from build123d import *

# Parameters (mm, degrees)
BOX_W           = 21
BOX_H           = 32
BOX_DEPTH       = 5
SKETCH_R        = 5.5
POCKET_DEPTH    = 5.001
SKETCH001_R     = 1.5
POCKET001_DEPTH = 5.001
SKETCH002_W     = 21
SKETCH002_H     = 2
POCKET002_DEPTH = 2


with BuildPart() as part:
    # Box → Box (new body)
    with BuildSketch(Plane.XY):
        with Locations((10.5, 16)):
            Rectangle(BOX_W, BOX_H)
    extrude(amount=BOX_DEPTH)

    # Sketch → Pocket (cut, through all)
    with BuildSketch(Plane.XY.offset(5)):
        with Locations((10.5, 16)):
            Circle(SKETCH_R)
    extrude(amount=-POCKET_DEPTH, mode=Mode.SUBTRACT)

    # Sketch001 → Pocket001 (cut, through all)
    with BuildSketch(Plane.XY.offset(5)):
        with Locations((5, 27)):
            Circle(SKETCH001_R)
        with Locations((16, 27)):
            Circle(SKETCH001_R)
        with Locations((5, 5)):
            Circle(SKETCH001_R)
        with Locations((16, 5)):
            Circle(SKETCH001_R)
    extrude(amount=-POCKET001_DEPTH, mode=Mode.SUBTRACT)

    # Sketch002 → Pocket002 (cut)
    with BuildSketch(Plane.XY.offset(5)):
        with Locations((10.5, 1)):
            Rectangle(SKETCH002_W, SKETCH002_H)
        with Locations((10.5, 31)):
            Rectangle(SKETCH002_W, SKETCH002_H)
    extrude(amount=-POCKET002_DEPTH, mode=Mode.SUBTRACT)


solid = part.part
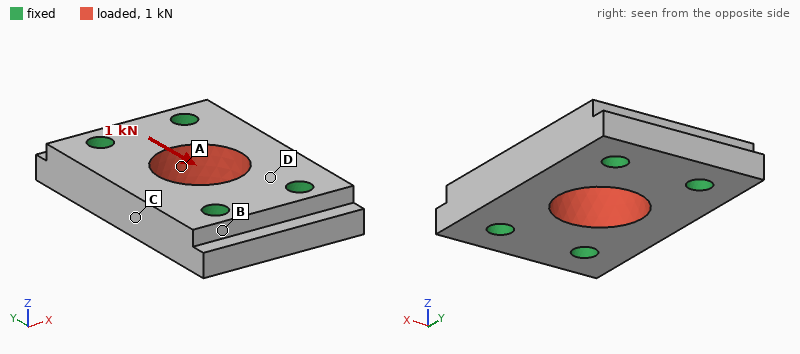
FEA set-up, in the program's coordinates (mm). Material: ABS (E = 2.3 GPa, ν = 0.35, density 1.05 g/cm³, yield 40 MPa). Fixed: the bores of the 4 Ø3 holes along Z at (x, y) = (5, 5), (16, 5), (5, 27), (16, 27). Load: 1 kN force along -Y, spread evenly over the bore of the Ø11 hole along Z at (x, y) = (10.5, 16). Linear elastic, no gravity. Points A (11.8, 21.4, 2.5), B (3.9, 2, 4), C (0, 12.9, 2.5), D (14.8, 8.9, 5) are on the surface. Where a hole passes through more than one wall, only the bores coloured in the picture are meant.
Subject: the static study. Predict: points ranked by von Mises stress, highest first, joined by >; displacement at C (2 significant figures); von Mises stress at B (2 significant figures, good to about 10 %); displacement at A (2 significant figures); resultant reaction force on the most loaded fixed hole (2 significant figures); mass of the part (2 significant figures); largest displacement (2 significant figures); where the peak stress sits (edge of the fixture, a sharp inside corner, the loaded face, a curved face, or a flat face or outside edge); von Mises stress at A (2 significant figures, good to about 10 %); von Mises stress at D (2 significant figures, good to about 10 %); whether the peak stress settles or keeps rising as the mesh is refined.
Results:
D > A > B > C
11 µm
2.5 MPa
18 µm
260 N
2.7 g
27 µm
edge of the fixture
5.3 MPa
7.6 MPa
keeps rising
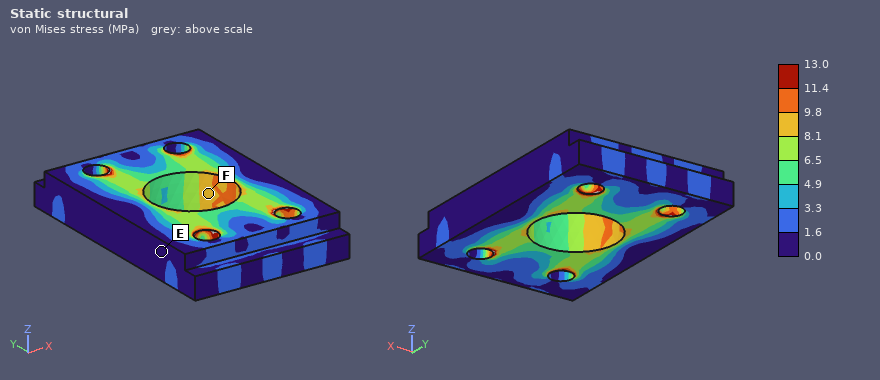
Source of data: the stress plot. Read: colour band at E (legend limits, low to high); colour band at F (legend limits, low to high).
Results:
0.0 to 1.6 MPa
8.1 to 9.8 MPa
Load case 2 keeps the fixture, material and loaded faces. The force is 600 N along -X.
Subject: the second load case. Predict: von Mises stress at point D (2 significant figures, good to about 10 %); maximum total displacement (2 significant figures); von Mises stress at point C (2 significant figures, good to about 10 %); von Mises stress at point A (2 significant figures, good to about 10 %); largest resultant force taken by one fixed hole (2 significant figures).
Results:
5.1 MPa
46 µm
5.4 MPa
7.9 MPa
160 N
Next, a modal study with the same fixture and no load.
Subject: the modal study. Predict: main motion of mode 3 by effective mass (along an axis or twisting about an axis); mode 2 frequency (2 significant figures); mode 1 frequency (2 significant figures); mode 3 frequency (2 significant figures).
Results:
along X
14 kHz
14 kHz
20 kHz
